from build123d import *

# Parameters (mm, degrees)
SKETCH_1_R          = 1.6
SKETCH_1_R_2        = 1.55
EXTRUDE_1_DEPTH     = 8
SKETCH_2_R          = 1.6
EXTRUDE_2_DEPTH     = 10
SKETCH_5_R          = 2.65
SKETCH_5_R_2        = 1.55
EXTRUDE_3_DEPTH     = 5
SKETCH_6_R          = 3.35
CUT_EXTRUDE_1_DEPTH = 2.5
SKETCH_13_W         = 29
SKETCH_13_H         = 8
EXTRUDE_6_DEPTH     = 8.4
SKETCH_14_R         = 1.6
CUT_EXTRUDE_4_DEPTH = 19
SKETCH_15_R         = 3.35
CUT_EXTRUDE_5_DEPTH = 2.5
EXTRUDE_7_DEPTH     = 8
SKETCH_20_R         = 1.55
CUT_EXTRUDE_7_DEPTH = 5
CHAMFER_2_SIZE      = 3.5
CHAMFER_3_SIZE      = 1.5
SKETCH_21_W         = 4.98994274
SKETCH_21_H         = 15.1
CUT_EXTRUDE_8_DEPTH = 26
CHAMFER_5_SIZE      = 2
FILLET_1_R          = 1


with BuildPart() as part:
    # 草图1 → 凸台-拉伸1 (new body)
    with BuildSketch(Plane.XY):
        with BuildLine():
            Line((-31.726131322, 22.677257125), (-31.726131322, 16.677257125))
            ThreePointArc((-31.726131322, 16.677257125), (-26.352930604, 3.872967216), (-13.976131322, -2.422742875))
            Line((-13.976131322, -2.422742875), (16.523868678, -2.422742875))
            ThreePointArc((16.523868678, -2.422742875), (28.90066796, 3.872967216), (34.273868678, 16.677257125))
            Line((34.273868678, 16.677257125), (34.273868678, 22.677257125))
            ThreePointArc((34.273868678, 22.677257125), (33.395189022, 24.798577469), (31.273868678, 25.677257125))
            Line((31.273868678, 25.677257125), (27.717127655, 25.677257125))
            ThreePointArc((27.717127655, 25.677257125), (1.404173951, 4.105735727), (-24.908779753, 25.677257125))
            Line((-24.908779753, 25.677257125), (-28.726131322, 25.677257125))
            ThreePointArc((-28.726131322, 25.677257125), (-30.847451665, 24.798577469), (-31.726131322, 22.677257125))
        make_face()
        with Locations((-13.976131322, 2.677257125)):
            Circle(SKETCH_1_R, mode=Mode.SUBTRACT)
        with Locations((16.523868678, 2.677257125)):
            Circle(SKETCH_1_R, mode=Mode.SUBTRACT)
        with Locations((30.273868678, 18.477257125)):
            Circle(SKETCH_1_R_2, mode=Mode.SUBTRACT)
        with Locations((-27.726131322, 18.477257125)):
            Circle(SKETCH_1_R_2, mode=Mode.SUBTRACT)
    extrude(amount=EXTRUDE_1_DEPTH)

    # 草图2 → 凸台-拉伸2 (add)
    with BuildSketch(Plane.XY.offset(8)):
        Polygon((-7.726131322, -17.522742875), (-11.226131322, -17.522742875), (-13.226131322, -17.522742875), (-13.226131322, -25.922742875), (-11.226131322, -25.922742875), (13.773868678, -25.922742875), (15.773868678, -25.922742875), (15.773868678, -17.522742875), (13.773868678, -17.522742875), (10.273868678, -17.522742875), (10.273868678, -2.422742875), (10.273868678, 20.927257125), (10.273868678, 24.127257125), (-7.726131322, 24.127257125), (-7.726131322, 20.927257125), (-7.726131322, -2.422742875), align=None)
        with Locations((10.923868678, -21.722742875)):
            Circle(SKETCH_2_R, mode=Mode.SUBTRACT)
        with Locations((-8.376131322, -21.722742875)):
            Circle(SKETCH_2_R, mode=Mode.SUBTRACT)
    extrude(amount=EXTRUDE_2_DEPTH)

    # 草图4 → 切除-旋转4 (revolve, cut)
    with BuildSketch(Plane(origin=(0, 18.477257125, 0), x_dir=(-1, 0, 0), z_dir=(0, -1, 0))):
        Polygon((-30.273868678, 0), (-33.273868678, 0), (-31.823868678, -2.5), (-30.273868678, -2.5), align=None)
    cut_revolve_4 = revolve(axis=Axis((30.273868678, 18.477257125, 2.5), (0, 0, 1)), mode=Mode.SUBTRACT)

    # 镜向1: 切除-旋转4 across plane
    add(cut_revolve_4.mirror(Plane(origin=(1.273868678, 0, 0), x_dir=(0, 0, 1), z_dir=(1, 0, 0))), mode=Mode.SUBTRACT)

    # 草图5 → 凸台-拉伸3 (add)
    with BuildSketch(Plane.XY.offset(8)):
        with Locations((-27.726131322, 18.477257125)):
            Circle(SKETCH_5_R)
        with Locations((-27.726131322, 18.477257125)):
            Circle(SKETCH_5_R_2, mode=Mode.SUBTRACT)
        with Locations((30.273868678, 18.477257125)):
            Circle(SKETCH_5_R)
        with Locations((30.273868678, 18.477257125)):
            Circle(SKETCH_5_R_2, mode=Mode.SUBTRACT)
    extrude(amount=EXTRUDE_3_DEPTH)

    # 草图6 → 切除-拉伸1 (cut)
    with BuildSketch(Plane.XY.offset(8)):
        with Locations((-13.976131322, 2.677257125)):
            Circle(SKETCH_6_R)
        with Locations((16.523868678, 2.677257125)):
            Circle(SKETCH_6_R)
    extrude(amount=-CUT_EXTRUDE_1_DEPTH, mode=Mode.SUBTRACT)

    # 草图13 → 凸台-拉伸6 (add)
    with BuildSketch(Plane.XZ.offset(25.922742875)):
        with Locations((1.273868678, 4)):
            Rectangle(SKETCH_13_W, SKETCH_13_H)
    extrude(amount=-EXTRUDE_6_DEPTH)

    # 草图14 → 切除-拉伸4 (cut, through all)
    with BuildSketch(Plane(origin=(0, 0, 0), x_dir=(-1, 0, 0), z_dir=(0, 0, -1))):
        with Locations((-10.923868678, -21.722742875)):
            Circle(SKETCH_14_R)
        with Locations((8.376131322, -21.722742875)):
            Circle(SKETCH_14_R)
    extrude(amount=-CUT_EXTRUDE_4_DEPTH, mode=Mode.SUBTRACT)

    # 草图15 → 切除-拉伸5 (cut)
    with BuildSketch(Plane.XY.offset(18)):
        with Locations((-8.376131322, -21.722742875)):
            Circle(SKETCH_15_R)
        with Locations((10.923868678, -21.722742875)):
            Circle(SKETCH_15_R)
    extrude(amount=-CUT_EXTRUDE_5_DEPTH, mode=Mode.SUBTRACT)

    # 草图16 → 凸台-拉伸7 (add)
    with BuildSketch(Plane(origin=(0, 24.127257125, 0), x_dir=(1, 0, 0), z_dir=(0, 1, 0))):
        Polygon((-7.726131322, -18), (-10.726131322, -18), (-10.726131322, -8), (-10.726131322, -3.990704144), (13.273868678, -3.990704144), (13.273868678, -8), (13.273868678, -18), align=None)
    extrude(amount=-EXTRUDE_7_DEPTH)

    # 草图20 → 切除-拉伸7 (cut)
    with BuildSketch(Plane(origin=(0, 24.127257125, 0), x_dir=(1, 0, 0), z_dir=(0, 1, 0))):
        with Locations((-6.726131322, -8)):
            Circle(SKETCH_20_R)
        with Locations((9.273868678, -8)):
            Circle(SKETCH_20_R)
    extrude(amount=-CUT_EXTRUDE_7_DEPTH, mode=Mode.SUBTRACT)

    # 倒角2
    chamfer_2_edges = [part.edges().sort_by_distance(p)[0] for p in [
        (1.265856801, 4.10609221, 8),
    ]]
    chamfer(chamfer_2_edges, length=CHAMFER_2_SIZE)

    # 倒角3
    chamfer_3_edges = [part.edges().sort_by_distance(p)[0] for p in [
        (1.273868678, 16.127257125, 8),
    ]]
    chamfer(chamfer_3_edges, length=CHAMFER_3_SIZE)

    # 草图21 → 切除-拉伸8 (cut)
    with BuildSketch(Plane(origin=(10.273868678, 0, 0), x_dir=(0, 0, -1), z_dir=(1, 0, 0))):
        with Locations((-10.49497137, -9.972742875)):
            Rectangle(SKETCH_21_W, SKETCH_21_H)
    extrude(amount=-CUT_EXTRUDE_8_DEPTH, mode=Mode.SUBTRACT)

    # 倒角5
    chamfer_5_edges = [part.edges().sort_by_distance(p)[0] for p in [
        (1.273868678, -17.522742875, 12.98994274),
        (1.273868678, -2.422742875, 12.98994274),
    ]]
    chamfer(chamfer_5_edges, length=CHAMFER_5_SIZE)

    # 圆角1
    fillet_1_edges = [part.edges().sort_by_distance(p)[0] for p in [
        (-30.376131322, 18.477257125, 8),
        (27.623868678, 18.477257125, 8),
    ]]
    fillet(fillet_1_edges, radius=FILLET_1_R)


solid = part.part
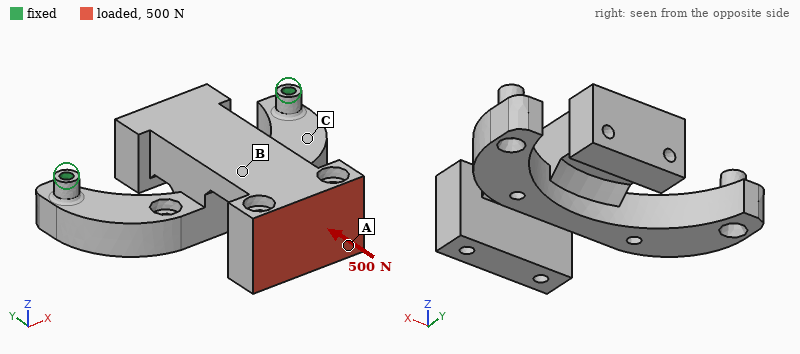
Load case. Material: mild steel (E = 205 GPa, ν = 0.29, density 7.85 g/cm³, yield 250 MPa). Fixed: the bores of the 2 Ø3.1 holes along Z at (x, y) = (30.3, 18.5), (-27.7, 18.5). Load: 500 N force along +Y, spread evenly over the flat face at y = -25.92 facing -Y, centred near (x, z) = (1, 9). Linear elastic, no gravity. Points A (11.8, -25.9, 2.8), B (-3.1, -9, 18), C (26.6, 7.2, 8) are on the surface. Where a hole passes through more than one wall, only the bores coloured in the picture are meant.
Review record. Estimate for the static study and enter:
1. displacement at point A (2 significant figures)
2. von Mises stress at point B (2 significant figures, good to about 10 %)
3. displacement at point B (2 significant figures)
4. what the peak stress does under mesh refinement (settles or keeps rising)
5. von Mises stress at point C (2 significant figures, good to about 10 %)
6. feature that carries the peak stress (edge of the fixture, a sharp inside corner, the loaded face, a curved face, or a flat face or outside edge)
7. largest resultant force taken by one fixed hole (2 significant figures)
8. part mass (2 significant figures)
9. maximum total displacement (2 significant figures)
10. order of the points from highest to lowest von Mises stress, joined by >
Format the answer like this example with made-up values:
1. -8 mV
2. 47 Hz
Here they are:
1. 20 µm
2. 34 MPa
3. 13 µm
4. keeps rising
5. 11 MPa
6. a sharp inside corner
7. 380 N
8. 140 g
9. 22 µm
10. B > C > A
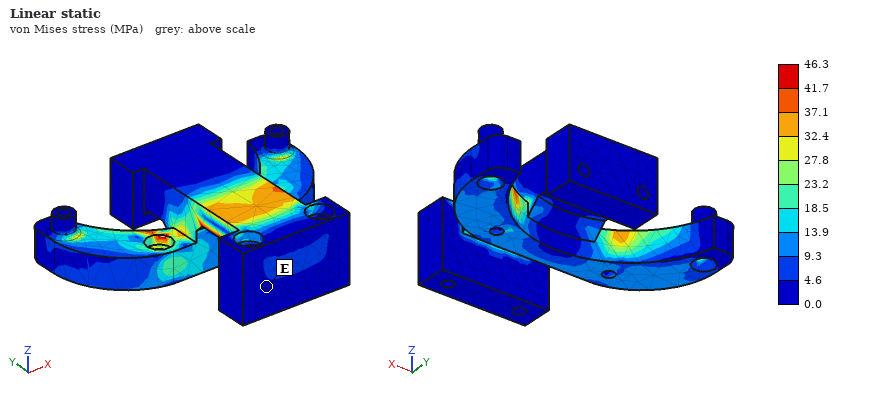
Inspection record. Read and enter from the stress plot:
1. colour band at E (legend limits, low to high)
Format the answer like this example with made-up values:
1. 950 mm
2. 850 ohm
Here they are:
1. 0.0 to 4.6 MPa
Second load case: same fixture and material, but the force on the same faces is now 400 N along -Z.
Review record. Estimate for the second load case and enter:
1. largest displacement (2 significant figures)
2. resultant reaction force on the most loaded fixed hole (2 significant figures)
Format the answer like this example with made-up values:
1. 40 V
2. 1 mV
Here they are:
1. 0.18 mm
2. 210 N
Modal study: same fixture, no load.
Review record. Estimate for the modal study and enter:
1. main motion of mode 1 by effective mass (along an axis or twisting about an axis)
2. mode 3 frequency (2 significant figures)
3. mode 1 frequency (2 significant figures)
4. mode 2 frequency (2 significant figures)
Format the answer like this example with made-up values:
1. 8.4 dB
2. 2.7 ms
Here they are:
1. along Z
2. 3500 Hz
3. 1400 Hz
4. 3400 Hz
